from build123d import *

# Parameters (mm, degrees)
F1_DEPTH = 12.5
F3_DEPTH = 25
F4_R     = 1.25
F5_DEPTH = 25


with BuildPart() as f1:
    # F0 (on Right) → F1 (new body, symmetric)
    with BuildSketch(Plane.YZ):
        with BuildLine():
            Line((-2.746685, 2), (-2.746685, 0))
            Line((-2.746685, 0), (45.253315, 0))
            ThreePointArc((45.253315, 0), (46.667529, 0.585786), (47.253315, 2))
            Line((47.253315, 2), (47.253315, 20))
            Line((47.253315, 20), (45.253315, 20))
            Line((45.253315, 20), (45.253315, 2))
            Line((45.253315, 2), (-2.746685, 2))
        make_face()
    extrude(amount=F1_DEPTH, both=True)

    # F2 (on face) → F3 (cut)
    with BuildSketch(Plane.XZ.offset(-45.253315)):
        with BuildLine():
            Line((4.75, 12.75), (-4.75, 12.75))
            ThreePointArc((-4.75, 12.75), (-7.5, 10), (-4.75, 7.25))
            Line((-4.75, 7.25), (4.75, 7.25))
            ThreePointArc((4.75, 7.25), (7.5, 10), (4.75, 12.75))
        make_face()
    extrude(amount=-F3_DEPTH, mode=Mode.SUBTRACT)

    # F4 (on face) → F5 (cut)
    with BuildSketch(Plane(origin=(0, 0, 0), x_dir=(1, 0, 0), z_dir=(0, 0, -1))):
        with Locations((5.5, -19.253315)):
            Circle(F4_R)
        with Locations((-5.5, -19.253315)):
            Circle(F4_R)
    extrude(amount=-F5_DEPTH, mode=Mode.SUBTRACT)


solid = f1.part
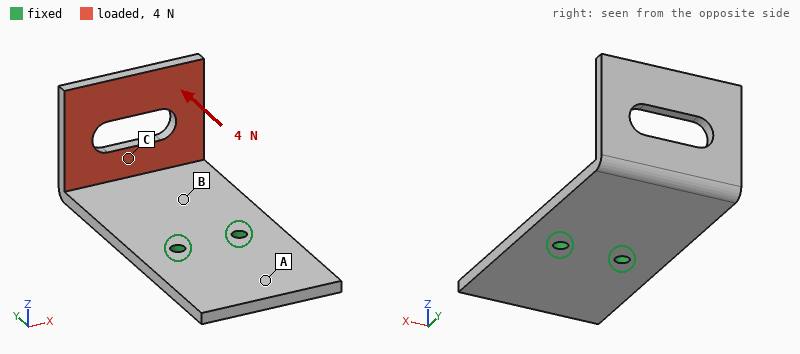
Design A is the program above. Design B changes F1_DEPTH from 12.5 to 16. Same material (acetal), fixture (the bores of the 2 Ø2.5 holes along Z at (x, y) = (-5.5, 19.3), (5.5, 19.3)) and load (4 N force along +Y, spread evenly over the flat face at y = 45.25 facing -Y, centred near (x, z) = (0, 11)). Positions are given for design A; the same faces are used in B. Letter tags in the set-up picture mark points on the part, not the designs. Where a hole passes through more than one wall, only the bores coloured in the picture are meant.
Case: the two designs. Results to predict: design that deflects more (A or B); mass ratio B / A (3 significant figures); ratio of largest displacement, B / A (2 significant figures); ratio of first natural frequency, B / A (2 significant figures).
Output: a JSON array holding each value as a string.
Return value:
["A", "1.29", "0.77", "0.97"]
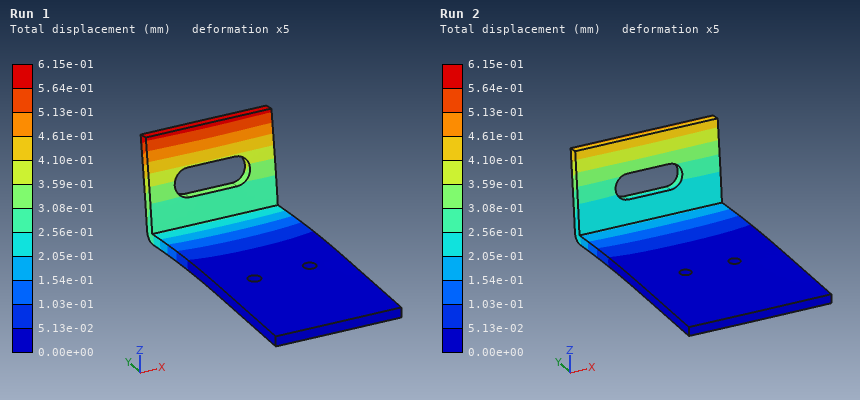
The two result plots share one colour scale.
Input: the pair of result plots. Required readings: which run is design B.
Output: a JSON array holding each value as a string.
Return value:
["Run 2"]
